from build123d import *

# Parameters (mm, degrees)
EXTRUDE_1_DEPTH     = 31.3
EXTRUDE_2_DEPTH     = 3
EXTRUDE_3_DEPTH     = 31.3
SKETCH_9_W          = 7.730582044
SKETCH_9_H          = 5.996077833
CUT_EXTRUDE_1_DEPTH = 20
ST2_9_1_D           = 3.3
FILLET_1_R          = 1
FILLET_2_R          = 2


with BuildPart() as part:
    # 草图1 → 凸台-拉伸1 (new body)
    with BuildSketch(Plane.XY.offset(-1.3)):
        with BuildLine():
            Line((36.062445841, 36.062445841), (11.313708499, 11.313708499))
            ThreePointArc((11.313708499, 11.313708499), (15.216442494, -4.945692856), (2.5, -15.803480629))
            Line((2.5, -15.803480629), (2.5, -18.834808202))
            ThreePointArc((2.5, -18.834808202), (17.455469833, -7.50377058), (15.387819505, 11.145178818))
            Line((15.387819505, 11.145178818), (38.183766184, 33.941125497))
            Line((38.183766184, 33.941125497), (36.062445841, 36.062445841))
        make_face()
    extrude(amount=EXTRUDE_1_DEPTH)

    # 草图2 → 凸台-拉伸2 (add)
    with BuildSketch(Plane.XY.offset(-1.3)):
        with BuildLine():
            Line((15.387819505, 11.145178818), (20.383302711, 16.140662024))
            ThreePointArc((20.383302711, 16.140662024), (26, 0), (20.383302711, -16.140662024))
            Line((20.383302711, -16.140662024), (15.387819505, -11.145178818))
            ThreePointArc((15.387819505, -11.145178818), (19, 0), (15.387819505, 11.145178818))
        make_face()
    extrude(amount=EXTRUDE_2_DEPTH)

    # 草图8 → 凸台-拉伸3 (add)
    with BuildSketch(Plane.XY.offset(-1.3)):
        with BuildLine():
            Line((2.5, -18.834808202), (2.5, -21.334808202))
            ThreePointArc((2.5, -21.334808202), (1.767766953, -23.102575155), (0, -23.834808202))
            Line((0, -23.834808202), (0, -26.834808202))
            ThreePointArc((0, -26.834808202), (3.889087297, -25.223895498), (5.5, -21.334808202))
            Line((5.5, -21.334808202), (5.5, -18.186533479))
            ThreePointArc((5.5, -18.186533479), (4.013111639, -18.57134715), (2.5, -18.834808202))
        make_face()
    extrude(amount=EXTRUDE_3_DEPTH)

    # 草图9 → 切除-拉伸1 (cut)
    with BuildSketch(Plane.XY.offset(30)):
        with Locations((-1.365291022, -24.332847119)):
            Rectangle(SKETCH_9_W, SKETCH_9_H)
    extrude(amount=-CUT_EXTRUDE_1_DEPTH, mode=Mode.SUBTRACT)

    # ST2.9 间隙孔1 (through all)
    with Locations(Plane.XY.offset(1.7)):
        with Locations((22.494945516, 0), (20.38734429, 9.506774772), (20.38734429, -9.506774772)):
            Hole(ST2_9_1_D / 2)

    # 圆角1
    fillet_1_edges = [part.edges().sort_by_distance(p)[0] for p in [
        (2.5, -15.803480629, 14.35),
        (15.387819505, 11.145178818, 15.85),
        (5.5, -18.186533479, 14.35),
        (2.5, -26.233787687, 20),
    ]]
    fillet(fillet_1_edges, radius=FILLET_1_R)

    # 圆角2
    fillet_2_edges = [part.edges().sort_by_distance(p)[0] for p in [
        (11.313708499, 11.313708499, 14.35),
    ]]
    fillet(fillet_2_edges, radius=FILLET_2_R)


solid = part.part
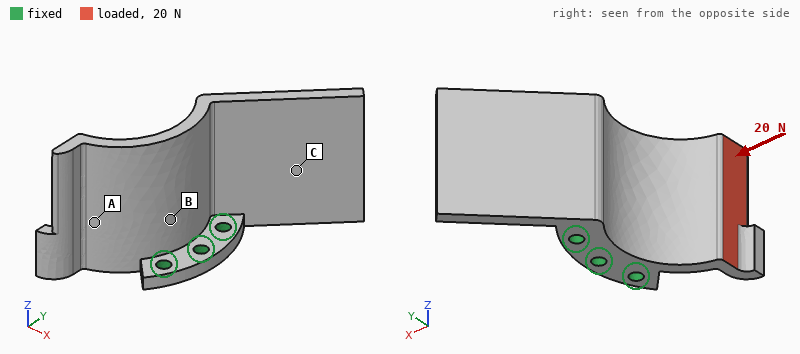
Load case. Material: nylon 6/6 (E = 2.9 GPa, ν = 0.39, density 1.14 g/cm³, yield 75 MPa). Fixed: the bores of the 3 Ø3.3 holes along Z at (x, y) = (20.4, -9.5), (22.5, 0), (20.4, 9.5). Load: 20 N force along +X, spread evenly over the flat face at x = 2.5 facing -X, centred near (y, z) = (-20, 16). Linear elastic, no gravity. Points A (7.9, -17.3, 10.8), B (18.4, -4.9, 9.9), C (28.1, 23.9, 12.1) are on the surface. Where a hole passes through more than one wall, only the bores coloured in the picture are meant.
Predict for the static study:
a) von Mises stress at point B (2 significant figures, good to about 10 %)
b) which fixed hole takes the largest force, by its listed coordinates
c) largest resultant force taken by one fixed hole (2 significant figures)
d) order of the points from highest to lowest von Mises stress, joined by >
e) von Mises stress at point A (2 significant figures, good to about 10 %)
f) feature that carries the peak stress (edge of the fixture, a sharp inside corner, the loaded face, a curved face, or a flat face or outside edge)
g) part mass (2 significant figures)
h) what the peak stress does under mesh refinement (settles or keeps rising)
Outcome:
4.9 MPa
(20.4, -9.5)
30 N
B > A > C
2.3 MPa
edge of the fixture
8.9 g
keeps rising
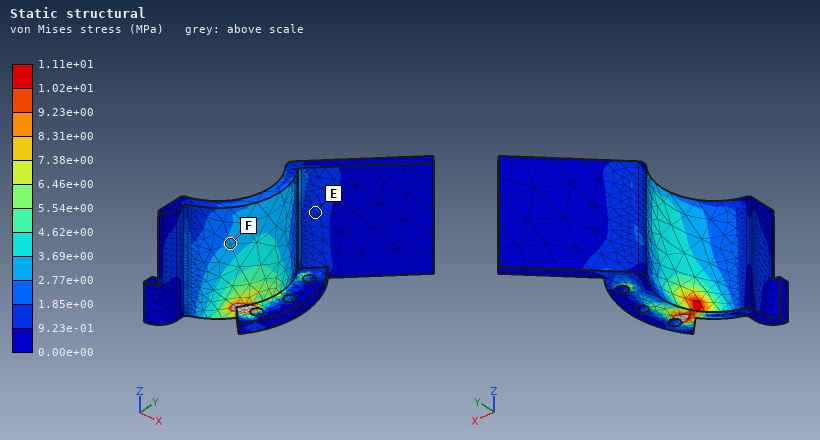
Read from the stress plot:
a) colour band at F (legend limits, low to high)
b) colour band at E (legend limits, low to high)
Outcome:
2.77e+00 to 3.69e+00 MPa
9.23e-01 to 1.85e+00 MPa
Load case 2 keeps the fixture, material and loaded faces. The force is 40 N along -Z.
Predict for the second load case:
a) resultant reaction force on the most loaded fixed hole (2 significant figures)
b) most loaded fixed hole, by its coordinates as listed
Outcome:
78 N
(20.4, -9.5)
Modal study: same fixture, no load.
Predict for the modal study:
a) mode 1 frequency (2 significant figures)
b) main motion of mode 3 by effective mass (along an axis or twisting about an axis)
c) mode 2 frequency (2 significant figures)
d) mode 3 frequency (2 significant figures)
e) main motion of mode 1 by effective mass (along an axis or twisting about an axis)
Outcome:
530 Hz
along Y
630 Hz
920 Hz
along X
